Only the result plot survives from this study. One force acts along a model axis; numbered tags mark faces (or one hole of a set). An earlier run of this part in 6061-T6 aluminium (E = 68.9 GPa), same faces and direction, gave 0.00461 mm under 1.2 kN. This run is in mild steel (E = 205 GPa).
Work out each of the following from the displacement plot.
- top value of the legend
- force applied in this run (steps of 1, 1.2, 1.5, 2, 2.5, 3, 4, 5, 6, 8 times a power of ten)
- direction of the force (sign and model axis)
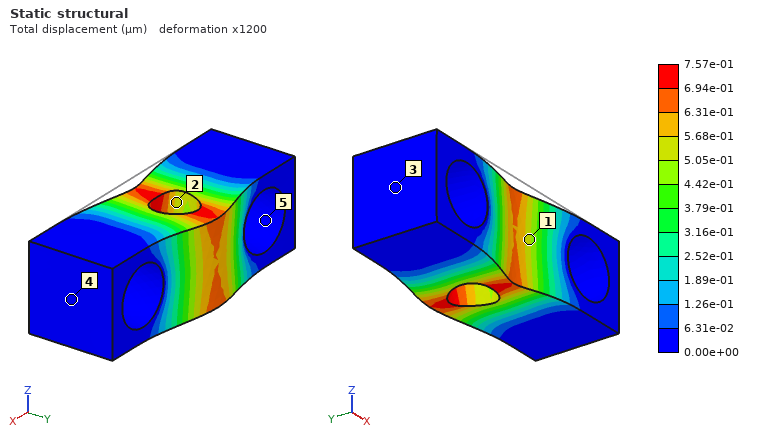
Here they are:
7.57e-01 µm
600 N
+Y
